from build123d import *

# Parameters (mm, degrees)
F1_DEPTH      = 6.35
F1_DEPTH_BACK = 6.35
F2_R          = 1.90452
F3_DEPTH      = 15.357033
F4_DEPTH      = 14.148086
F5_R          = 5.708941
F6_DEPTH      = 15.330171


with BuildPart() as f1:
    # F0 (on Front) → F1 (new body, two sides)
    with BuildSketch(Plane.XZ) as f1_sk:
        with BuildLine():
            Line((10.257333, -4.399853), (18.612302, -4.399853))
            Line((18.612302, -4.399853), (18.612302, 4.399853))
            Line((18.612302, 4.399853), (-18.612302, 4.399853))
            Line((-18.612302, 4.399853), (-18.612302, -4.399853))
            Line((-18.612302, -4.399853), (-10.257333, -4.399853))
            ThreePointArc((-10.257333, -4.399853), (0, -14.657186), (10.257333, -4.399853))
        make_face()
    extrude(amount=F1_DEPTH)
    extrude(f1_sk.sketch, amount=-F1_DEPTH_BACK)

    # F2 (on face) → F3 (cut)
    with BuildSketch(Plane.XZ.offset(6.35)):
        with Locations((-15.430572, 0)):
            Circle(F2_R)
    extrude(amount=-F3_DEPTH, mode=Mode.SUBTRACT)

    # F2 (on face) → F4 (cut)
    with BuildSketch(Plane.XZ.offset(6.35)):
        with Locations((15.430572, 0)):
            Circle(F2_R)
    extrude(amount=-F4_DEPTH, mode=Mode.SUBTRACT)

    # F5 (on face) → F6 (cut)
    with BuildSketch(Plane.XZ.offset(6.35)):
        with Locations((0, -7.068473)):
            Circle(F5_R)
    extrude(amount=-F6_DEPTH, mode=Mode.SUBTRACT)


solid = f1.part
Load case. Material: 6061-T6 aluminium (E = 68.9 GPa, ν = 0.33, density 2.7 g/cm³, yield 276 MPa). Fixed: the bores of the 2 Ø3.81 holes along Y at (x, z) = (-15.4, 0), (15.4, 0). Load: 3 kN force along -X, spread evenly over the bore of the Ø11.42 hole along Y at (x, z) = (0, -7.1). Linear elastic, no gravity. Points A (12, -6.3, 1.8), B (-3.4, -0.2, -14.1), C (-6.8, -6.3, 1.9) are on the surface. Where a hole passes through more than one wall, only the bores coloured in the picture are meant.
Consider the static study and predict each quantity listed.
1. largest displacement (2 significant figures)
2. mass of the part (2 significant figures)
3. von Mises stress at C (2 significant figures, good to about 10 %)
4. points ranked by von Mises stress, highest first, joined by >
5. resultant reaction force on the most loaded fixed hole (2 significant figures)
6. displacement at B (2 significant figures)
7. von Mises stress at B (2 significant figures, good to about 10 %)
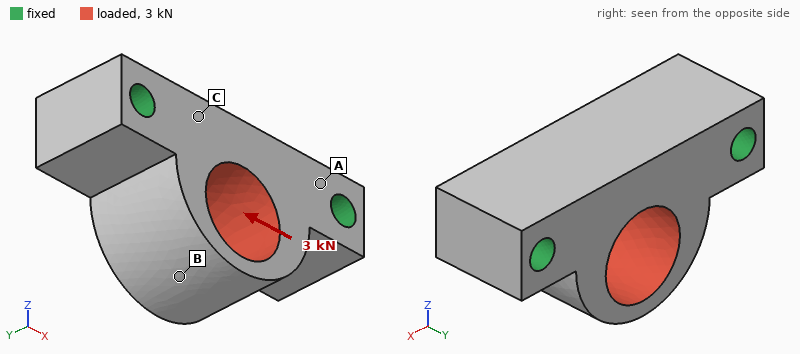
22 µm
13 g
13 MPa
B > C > A
1.7 kN
20 µm
47 MPa
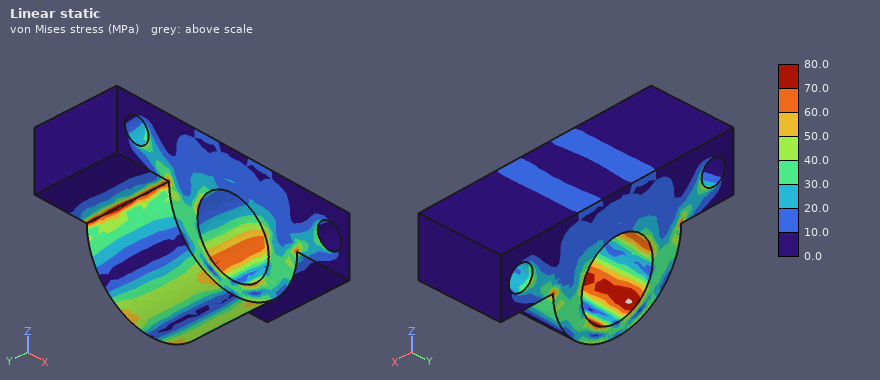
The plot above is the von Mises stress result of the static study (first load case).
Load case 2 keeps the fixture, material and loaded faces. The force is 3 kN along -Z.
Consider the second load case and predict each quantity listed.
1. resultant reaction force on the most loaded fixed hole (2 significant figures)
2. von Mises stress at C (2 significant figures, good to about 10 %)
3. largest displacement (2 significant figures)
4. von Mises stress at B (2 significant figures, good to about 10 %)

1.5 kN
15 MPa
12 µm
19 MPa
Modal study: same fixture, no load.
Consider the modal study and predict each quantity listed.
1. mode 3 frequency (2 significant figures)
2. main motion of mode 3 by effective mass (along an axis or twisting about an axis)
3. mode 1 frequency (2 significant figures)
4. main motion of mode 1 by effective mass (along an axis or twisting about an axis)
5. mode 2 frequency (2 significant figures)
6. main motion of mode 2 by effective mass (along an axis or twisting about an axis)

34 kHz
along X
25 kHz
along Y
31 kHz
along Z
